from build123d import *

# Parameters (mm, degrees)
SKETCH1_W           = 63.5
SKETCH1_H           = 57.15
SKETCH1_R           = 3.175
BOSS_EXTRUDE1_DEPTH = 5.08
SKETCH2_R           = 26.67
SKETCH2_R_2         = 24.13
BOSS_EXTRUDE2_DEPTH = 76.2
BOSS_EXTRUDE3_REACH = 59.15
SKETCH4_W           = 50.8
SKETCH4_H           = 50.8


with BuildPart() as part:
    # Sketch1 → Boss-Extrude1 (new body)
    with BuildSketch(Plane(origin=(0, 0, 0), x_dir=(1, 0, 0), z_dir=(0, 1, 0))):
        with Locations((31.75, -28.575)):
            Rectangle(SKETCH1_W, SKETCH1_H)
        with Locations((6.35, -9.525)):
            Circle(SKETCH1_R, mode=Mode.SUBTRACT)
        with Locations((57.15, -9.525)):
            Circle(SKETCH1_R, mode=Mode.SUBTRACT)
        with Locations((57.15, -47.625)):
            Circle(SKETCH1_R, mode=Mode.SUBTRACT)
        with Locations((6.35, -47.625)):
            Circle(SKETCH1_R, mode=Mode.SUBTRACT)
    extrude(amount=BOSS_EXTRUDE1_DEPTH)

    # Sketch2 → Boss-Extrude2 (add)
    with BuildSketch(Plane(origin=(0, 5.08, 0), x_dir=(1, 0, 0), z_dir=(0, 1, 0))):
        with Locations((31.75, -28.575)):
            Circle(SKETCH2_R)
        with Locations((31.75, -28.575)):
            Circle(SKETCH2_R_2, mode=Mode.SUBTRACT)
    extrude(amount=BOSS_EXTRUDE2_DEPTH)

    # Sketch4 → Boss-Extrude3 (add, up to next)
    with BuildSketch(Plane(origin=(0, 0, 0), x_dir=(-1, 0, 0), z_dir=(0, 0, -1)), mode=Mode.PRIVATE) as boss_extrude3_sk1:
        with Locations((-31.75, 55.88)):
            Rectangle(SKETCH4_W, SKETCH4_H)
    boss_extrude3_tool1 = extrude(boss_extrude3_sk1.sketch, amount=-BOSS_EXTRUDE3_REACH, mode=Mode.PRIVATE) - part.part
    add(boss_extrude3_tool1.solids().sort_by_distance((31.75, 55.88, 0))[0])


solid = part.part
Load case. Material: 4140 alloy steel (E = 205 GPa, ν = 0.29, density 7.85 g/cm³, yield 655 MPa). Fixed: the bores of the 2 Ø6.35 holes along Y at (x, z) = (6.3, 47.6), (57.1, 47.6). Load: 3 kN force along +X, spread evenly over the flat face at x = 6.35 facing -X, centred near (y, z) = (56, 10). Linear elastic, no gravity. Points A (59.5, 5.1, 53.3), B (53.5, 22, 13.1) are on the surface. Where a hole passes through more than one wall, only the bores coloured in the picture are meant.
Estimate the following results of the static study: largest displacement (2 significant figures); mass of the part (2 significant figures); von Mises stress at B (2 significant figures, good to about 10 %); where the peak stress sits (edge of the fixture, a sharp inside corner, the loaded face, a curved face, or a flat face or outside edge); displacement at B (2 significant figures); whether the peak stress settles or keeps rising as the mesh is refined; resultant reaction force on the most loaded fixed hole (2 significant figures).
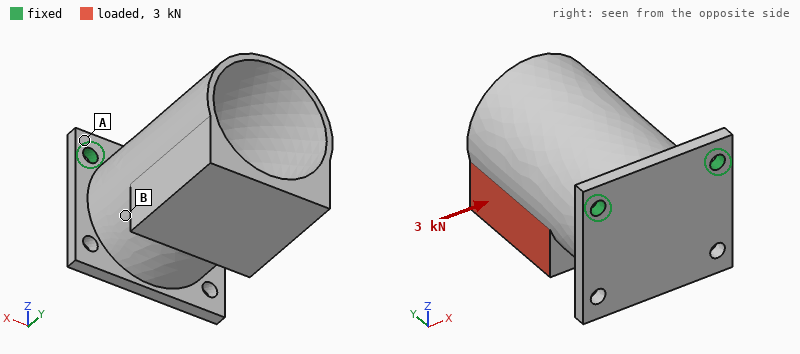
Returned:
0.12 mm
520 g
25 MPa
edge of the fixture
0.039 mm
keeps rising
4.3 kN
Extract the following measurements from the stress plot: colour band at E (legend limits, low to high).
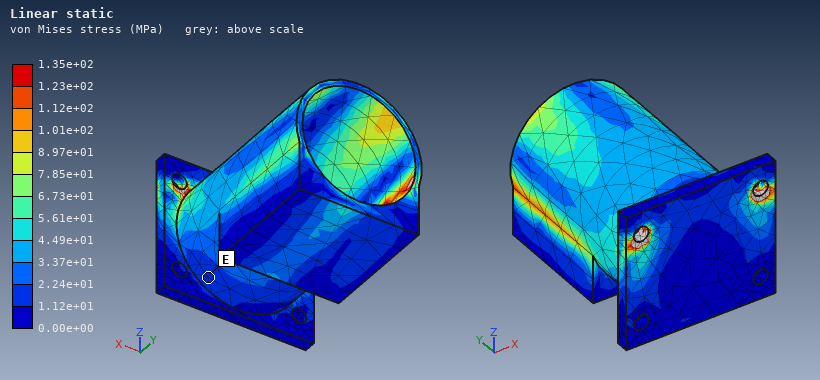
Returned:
1.12e+01 to 2.24e+01 MPa
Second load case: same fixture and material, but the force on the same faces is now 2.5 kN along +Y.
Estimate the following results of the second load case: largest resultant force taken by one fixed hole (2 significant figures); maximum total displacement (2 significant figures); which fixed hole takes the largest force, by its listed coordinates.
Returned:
2.6 kN
0.41 mm
(6.3, 47.6)
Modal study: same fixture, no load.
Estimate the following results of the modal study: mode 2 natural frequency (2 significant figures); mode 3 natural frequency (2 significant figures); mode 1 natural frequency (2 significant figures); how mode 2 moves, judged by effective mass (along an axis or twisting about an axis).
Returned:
1900 Hz
3800 Hz
600 Hz
along X
